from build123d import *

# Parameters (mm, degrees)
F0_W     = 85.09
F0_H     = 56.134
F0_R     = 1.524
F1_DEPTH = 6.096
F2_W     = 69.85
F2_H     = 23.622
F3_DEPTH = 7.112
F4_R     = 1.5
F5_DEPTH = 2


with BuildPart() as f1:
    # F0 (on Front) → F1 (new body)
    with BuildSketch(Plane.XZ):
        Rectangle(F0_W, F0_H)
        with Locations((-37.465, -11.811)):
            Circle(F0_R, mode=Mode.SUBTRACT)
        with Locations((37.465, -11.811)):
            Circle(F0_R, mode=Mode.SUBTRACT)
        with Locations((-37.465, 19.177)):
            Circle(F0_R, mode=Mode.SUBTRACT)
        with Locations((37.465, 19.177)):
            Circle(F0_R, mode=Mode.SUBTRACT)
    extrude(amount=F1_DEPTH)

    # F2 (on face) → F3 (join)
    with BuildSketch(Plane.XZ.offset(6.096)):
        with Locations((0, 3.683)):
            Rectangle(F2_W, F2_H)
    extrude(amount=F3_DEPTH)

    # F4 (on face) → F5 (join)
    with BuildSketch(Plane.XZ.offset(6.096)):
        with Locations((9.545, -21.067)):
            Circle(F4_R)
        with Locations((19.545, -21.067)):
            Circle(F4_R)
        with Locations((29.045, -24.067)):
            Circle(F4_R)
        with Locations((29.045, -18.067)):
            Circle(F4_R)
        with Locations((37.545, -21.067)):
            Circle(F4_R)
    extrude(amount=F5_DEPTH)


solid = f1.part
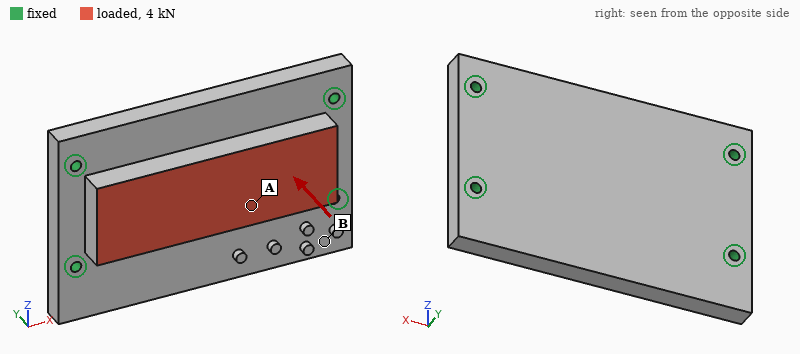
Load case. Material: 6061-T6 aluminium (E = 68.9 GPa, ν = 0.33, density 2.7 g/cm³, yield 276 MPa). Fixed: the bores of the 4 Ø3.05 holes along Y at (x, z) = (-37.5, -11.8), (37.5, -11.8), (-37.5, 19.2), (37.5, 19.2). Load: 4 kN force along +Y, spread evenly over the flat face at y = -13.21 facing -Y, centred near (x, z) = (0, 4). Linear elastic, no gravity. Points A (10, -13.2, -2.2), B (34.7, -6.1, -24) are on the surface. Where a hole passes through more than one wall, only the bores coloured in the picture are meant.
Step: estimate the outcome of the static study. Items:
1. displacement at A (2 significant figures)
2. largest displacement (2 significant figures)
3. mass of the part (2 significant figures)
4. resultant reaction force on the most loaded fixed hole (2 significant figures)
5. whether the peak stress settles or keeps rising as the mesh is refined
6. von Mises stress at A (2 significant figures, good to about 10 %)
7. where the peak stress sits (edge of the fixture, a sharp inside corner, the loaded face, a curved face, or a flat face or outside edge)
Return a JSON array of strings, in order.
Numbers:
["33 µm", "39 µm", "110 g", "1.3 kN", "keeps rising", "26 MPa", "edge of the fixture"]
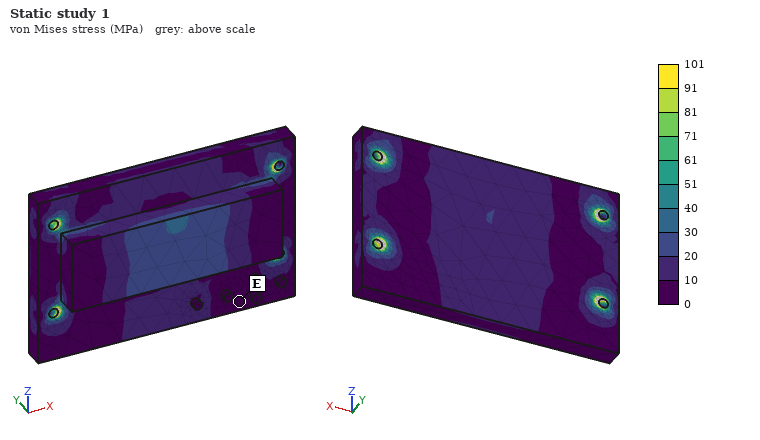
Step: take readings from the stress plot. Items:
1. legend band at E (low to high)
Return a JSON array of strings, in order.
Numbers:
["0 to 10 MPa"]
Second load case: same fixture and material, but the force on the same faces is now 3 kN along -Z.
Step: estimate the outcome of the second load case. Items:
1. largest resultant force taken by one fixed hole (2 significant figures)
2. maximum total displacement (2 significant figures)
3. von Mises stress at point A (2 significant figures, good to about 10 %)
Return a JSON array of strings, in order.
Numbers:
["1.0 kN", "16 µm", "6.4 MPa"]
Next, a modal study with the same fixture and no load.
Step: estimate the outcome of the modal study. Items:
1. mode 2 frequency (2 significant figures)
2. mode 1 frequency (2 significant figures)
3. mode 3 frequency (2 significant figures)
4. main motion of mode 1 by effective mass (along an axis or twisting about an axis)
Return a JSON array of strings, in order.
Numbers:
["7800 Hz", "5700 Hz", "13 kHz", "along Y"]
